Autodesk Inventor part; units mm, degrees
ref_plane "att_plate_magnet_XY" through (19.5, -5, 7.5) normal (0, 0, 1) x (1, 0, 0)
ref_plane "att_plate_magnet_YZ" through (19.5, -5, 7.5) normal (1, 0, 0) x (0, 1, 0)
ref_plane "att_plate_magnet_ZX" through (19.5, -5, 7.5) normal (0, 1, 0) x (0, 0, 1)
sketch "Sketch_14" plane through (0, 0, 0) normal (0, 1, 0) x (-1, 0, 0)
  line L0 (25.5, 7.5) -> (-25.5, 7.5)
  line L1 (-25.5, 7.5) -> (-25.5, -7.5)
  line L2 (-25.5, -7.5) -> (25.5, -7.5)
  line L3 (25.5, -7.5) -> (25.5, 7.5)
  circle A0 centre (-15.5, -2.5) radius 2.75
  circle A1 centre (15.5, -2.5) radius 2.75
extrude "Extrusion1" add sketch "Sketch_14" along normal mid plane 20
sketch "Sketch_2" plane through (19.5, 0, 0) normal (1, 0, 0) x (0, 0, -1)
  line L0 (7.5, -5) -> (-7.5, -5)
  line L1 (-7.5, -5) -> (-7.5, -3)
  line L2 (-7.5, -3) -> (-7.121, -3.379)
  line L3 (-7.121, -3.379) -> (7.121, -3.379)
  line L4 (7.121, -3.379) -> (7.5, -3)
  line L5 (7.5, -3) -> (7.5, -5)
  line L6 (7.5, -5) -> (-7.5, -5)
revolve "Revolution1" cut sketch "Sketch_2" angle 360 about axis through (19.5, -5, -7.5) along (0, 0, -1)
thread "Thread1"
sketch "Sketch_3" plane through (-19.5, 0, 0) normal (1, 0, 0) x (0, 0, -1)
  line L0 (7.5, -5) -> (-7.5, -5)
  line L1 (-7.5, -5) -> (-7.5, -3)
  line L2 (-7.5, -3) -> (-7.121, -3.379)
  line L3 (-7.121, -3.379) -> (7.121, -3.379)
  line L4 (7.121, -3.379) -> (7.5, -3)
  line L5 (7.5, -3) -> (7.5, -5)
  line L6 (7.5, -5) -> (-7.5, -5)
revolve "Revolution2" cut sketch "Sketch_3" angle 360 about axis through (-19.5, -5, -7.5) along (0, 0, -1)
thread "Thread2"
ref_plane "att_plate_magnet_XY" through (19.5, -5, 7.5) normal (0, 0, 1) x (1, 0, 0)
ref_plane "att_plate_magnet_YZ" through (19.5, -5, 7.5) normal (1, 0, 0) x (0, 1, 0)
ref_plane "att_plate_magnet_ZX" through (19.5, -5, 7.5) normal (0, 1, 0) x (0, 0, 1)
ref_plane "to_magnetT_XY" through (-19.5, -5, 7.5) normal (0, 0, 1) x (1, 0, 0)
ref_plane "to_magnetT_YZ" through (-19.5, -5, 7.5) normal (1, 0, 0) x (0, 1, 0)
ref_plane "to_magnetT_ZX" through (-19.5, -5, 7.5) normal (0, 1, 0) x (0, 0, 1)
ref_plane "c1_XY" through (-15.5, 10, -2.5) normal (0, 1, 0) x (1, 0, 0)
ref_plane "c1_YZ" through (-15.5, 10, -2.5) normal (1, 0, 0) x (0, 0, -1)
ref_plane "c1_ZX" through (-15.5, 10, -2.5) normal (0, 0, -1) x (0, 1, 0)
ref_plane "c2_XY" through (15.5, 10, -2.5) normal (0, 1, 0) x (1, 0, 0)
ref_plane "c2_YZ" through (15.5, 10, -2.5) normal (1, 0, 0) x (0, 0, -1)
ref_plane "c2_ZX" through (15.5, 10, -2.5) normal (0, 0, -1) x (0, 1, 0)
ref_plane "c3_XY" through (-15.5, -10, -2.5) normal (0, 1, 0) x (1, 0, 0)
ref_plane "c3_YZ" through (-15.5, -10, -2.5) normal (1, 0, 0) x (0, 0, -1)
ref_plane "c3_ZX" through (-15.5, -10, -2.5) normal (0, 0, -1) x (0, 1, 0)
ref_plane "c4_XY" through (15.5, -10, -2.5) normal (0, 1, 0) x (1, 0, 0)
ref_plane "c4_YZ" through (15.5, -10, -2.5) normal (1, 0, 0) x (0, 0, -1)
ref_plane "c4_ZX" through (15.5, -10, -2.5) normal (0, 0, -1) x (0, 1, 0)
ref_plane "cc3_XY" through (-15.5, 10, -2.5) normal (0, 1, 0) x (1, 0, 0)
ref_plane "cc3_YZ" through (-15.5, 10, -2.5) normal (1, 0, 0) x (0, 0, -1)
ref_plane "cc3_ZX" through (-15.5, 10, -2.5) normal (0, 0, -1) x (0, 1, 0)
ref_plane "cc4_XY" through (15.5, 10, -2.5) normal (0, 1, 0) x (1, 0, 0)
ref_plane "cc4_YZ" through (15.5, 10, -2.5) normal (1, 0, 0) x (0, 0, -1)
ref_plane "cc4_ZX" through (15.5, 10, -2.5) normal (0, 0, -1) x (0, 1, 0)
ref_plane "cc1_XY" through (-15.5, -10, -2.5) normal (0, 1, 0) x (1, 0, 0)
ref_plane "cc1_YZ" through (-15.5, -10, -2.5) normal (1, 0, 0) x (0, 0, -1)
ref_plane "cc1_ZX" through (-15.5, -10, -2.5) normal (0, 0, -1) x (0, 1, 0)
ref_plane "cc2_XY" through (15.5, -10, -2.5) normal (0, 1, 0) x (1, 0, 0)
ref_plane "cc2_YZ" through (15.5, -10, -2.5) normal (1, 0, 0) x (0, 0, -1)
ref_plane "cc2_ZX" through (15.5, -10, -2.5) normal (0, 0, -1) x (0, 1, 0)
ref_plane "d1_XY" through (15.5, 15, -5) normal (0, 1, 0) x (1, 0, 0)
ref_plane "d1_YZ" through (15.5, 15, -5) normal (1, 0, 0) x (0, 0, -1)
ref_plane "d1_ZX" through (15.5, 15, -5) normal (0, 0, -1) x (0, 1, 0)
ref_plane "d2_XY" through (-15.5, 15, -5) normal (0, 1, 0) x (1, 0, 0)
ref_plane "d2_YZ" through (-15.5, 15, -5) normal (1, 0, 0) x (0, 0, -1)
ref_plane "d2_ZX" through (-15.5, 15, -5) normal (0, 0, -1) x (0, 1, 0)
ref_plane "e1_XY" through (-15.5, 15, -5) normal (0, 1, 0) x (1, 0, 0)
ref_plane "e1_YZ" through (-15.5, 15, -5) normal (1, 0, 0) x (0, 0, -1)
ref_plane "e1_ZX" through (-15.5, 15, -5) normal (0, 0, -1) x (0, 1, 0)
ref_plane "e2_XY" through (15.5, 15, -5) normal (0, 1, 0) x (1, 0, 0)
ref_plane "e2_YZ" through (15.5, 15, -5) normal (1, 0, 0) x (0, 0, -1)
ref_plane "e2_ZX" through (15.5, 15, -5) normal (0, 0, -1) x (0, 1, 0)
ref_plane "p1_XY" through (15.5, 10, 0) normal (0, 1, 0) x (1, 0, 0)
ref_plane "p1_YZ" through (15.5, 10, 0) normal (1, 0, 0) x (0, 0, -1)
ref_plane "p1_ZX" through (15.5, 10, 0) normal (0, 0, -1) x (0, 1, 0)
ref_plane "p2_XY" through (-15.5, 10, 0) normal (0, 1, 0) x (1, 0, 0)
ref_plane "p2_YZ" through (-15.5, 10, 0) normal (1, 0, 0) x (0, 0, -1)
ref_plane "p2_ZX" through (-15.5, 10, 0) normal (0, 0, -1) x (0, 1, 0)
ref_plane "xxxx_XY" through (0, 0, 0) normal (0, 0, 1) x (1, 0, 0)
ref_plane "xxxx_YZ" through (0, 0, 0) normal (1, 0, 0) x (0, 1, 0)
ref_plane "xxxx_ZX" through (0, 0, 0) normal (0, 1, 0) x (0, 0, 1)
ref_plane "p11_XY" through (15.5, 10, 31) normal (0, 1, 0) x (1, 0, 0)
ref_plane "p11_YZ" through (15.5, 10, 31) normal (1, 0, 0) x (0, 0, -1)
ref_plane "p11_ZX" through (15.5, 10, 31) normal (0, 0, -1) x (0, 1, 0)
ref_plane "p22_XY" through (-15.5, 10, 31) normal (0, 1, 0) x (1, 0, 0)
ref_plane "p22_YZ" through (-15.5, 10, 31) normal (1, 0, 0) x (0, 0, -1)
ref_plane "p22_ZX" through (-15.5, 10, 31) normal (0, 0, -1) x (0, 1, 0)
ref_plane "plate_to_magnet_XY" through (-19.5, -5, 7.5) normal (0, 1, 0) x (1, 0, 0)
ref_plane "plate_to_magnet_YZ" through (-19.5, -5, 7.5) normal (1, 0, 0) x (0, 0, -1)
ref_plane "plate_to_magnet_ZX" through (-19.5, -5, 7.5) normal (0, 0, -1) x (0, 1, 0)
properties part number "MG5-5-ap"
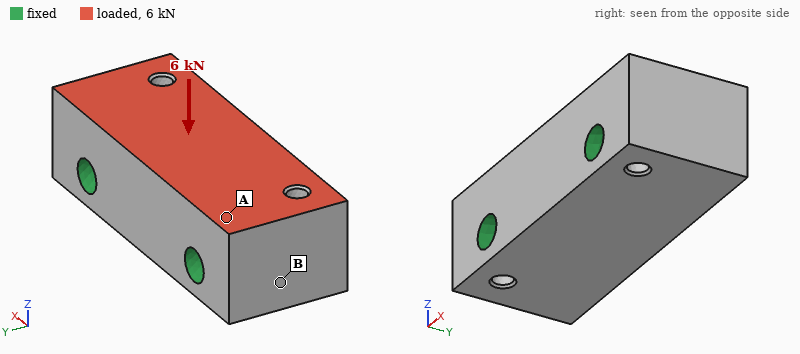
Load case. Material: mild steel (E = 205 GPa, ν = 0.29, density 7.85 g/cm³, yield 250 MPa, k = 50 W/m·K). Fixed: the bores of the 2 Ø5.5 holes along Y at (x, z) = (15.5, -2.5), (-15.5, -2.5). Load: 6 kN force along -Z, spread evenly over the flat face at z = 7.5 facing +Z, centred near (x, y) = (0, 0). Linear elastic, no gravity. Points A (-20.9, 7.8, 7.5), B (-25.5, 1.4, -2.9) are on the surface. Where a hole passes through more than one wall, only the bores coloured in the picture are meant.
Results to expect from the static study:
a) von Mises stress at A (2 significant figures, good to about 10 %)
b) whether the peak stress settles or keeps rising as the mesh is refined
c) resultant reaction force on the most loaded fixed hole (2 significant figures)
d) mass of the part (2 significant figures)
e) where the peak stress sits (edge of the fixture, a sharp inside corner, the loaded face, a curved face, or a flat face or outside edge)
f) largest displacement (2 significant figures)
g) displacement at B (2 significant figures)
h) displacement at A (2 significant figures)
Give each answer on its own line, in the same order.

7.5 MPa
keeps rising
3.0 kN
110 g
edge of the fixture
1.0 µm
0.33 µm
0.44 µm
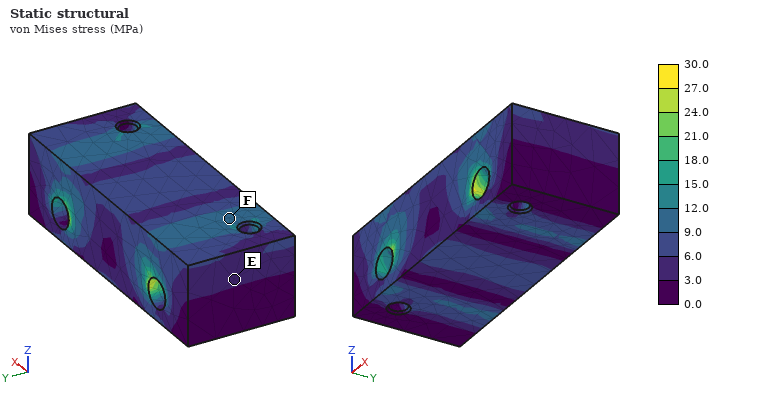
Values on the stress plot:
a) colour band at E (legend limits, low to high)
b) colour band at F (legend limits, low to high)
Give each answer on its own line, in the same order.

3.0 to 6.0 MPa
9.0 to 12.0 MPa
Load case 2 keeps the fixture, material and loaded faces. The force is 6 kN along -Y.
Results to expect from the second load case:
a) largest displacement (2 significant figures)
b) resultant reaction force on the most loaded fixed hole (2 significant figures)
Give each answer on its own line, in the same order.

2.9 µm
3.0 kN
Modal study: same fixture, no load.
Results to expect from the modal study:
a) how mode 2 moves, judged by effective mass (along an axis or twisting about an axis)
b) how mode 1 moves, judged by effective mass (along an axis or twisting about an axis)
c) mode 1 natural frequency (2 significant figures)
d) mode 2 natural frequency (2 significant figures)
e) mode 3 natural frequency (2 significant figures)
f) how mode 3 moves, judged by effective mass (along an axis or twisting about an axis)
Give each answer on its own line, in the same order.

along Y
along Z
39 kHz
43 kHz
50 kHz
along X
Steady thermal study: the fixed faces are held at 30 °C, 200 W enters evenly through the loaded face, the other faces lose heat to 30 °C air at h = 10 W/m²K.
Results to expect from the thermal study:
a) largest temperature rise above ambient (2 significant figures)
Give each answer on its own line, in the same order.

58 K
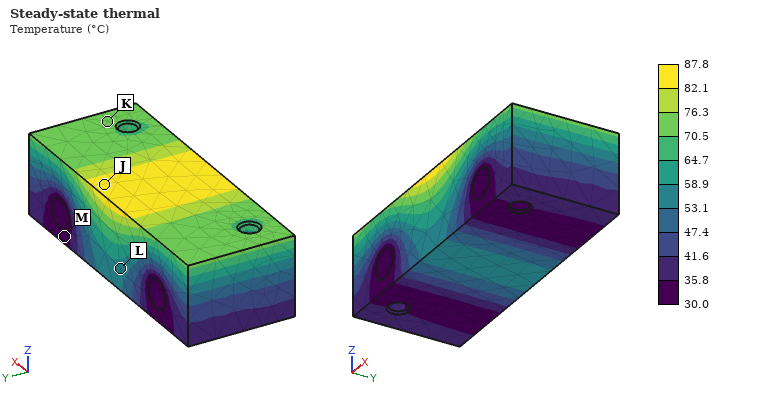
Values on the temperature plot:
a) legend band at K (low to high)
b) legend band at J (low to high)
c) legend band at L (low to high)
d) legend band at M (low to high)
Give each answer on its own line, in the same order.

70.5 to 76.3 °C
82.1 to 87.8 °C
53.1 to 58.9 °C
30.0 to 35.8 °C
